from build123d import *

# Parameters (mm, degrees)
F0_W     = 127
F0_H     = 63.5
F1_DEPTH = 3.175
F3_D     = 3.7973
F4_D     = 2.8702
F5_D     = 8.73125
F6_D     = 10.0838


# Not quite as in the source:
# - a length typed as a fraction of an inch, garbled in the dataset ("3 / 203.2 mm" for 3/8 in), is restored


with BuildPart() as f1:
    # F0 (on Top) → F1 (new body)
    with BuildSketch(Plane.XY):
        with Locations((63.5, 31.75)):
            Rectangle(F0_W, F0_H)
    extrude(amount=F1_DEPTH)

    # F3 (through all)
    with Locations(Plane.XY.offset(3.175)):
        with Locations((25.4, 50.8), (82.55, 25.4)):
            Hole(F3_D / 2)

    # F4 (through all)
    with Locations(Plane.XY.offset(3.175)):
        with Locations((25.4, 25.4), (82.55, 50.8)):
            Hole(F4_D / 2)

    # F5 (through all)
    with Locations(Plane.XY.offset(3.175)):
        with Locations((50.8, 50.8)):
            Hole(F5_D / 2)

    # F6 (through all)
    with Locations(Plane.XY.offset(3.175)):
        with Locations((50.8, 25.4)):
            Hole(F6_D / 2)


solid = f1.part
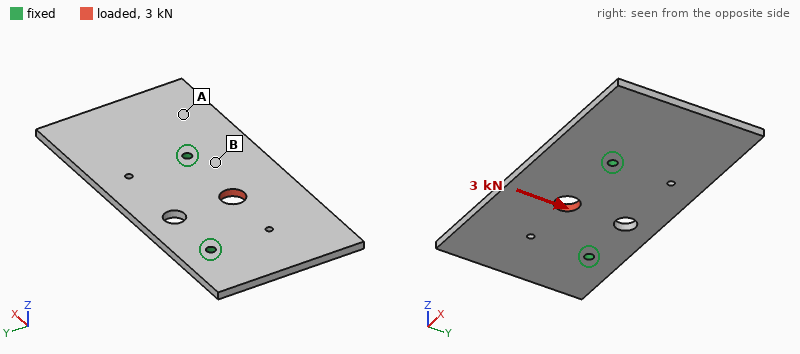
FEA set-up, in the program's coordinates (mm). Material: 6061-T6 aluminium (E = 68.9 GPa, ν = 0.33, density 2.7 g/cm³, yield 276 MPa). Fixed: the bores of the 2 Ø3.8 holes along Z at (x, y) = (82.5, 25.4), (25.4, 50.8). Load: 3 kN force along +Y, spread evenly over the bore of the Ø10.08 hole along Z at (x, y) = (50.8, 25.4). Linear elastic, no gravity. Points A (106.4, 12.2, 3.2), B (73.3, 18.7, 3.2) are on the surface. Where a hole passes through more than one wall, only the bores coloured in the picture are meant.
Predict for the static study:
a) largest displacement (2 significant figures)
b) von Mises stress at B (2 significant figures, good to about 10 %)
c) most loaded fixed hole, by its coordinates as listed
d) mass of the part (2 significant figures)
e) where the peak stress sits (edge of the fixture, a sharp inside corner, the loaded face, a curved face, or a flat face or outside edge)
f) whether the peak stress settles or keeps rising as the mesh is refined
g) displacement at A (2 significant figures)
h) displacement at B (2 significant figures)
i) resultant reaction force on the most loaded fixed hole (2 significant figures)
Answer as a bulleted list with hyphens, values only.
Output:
- 18 µm
- 16 MPa
- (25.4, 50.8)
- 68 g
- edge of the fixture
- keeps rising
- 3.8 µm
- 6.3 µm
- 1.7 kN
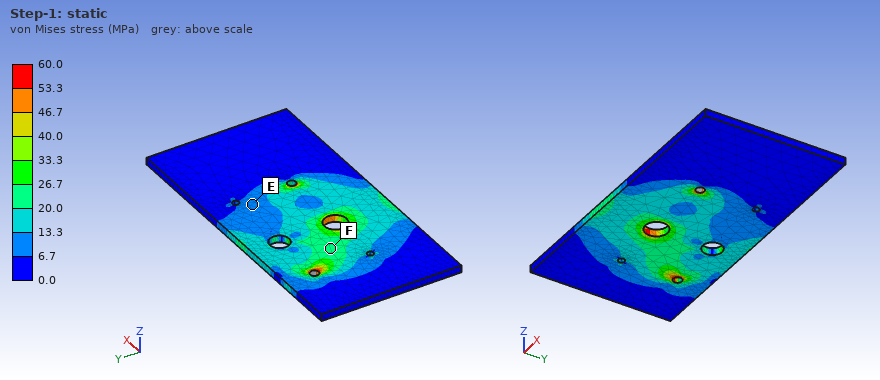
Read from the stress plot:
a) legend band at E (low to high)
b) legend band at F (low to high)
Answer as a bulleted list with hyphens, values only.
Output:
- 6.7 to 13.3 MPa
- 20.0 to 26.7 MPa
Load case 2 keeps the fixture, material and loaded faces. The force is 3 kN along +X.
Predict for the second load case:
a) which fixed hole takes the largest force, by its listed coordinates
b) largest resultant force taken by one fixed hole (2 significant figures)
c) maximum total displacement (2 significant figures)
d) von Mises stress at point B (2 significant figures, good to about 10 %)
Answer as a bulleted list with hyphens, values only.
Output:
- (82.5, 25.4)
- 2.0 kN
- 16 µm
- 24 MPa
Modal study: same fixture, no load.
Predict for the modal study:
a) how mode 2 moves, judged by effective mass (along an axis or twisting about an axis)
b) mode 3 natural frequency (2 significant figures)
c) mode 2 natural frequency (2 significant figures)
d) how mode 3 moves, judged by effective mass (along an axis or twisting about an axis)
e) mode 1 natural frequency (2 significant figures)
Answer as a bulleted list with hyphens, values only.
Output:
- along Z
- 1500 Hz
- 1200 Hz
- twisting about X
- 980 Hz
